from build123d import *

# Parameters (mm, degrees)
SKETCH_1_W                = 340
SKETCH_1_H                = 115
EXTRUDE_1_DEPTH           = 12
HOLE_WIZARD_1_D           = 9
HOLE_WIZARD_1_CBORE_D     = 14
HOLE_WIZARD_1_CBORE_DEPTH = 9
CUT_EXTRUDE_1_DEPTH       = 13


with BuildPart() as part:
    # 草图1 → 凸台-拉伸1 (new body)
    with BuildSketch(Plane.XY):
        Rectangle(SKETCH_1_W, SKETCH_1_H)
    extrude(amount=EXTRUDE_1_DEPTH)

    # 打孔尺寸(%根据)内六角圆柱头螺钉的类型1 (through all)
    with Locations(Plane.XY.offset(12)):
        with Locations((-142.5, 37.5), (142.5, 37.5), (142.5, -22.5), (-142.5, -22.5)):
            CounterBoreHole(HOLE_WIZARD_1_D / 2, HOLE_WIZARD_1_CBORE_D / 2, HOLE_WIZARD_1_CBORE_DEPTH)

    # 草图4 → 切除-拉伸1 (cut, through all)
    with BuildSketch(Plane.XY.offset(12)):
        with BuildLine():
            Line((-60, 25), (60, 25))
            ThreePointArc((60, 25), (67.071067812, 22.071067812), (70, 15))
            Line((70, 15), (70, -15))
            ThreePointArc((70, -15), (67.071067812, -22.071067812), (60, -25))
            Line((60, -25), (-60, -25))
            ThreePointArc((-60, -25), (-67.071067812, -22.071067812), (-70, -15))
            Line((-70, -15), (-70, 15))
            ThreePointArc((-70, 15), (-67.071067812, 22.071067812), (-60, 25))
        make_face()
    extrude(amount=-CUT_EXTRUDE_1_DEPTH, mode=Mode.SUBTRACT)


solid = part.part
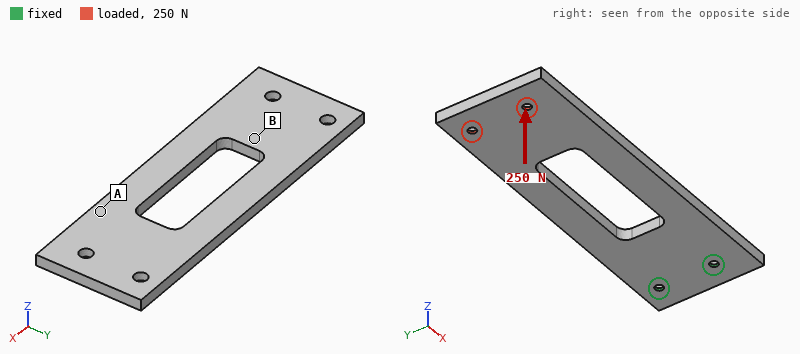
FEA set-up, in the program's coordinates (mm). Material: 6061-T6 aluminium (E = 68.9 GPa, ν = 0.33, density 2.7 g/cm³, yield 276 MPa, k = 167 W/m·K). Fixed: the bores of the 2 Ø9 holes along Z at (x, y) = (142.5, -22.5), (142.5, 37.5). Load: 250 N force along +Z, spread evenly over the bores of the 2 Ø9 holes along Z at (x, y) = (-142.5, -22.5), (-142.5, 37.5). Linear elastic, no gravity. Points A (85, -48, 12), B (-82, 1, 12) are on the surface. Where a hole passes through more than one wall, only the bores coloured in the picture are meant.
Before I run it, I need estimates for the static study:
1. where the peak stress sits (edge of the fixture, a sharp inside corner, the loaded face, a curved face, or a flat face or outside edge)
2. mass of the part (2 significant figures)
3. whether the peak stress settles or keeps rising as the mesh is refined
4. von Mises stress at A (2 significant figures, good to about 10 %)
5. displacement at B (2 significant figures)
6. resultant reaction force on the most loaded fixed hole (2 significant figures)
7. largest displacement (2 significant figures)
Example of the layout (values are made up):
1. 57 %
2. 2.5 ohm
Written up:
1. edge of the fixture
2. 1.0 kg
3. keeps rising
4. 25 MPa
5. 2.5 mm
6. 590 N
7. 4.0 mm
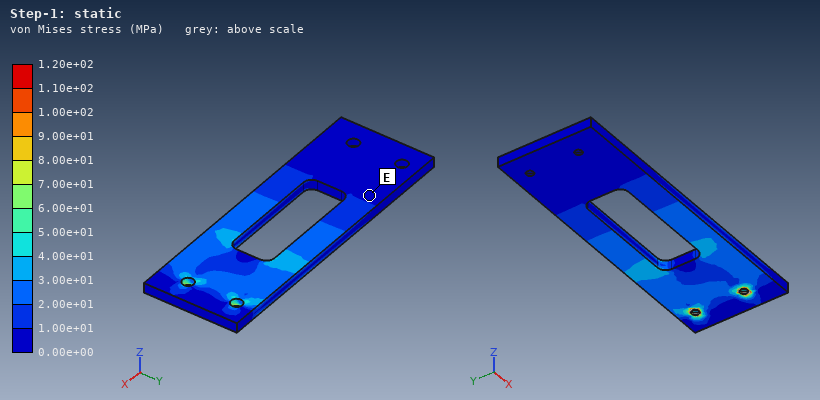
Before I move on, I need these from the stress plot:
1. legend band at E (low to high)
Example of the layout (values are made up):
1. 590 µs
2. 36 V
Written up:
1. 0.00e+00 to 1.00e+01 MPa
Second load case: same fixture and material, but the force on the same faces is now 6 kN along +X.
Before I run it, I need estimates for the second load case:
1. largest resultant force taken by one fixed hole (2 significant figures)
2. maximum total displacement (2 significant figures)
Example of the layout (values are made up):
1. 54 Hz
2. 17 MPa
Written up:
1. 3.0 kN
2. 1.6 mm
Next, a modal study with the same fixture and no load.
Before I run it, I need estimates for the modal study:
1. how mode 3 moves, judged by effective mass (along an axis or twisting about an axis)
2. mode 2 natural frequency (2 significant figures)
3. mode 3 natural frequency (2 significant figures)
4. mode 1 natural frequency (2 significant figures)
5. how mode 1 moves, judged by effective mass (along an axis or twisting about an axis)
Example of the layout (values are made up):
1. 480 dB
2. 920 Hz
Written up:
1. along Z
2. 420 Hz
3. 500 Hz
4. 72 Hz
5. along Z
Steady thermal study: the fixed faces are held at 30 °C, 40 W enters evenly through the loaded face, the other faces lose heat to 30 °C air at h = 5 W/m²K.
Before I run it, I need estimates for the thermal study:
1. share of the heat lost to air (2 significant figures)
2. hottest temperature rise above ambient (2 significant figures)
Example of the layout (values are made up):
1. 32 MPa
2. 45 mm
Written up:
1. 30 %
2. 64 K
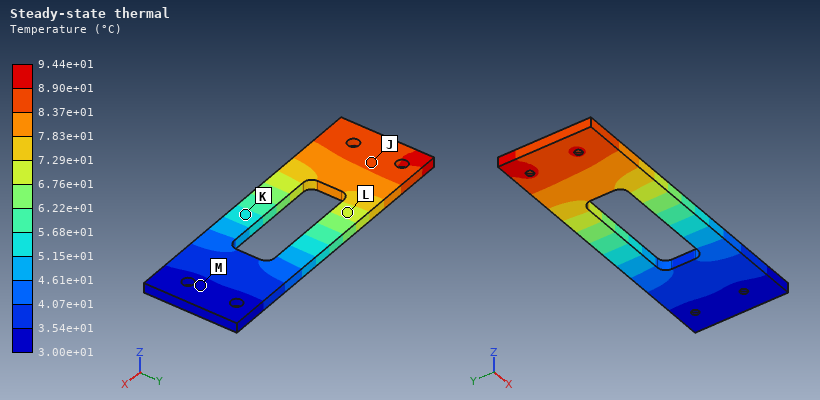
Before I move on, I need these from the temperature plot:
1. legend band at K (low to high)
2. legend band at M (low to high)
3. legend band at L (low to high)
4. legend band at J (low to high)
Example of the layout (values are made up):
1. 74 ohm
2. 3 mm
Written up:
1. 5.15e+01 to 5.68e+01 °C
2. 3.00e+01 to 3.54e+01 °C
3. 6.76e+01 to 7.29e+01 °C
4. 8.37e+01 to 8.90e+01 °C
